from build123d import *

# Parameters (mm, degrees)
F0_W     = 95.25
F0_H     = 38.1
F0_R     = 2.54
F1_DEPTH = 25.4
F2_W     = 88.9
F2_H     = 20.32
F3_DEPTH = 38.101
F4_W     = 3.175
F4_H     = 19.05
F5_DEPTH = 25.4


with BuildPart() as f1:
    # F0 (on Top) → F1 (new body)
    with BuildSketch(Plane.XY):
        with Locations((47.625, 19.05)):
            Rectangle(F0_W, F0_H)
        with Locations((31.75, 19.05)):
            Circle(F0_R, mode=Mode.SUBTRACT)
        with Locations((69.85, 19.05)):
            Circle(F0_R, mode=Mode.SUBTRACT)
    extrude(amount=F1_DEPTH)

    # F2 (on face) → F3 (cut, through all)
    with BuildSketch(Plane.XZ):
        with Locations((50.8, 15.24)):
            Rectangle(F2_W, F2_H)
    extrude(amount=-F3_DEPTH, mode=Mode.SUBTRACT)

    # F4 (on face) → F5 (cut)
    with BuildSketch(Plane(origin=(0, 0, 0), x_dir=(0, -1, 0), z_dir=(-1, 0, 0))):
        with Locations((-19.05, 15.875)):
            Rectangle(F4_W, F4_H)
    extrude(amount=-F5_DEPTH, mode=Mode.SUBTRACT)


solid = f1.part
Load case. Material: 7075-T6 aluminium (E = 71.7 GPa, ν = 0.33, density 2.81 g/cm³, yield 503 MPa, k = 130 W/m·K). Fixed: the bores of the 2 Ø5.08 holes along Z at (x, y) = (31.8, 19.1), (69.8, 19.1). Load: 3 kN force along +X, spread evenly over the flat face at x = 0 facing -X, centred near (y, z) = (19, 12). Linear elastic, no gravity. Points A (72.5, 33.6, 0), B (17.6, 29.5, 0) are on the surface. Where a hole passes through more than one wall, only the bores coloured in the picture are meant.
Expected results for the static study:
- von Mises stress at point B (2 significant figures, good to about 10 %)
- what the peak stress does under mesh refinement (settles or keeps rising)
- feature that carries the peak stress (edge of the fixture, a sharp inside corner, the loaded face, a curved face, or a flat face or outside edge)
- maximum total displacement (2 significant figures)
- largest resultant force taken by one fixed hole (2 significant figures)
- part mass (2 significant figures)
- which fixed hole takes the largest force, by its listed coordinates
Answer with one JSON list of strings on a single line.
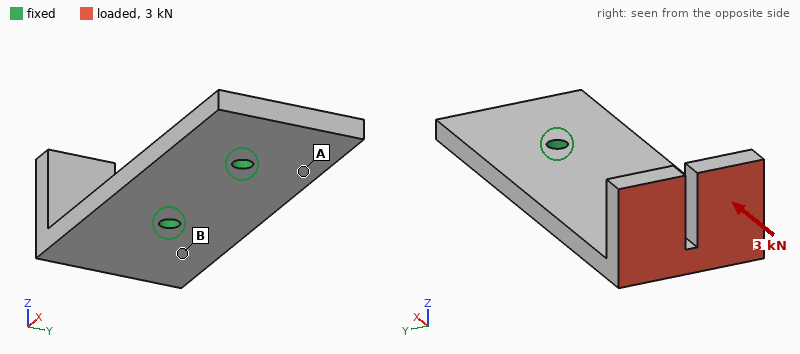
["150 MPa", "keeps rising", "edge of the fixture", "0.88 mm", "2.4 kN", "64 g", "(31.8, 19.1)"]
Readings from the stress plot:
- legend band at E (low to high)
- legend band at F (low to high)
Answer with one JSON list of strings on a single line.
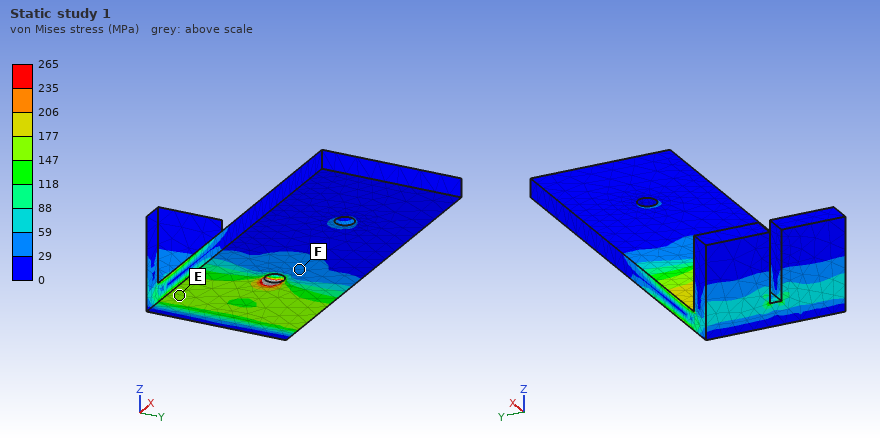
["147 to 177 MPa", "29 to 59 MPa"]
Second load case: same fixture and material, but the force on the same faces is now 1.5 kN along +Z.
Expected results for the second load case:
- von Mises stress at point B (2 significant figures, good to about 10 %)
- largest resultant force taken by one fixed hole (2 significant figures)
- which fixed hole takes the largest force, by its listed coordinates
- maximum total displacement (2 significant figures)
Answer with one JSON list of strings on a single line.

["150 MPa", "1.9 kN", "(31.8, 19.1)", "0.84 mm"]
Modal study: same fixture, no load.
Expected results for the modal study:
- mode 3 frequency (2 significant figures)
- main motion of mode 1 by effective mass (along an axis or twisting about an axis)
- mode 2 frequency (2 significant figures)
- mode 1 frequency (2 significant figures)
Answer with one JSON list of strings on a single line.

["5700 Hz", "along Z", "2800 Hz", "1900 Hz"]
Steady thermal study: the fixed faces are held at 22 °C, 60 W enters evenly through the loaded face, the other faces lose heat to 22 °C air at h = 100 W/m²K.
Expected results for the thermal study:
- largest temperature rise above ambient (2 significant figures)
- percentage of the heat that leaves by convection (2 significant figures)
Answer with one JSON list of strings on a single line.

["72 K", "32 %"]
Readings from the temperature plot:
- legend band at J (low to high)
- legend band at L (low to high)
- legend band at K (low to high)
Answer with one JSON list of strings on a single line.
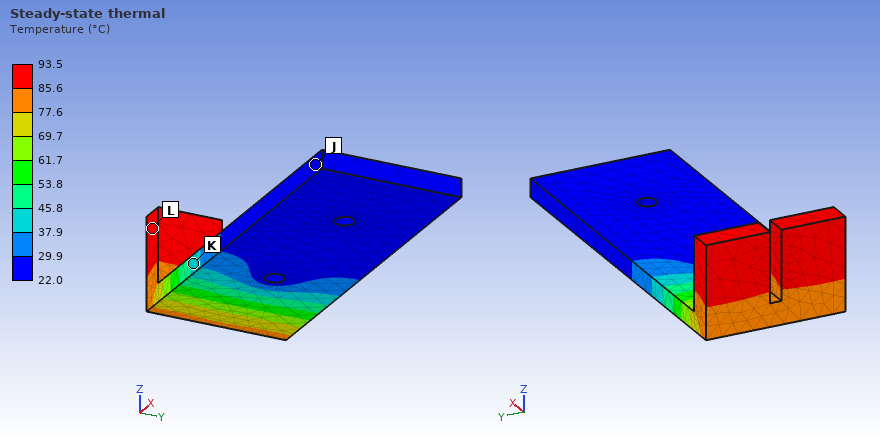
["22.0 to 29.9 °C", "85.6 to 93.5 °C", "37.9 to 45.8 °C"]
